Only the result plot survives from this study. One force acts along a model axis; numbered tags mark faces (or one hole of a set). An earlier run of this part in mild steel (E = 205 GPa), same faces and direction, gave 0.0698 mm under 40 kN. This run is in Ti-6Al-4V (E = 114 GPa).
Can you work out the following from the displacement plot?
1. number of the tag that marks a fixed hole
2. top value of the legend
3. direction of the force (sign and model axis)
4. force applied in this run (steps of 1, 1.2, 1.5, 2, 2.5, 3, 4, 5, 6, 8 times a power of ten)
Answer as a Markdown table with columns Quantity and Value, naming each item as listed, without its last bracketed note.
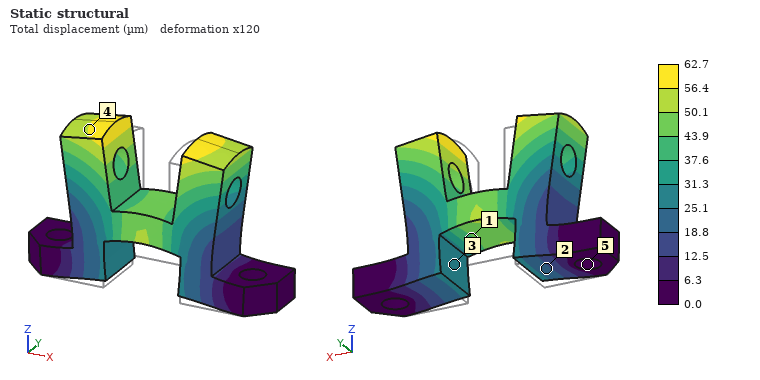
| Quantity | Value |
|---|---|
| number of the tag that marks a fixed hole | 5 |
| top value of the legend | 62.7 µm |
| direction of the force | +Z |
| force applied in this run | 20 kN |
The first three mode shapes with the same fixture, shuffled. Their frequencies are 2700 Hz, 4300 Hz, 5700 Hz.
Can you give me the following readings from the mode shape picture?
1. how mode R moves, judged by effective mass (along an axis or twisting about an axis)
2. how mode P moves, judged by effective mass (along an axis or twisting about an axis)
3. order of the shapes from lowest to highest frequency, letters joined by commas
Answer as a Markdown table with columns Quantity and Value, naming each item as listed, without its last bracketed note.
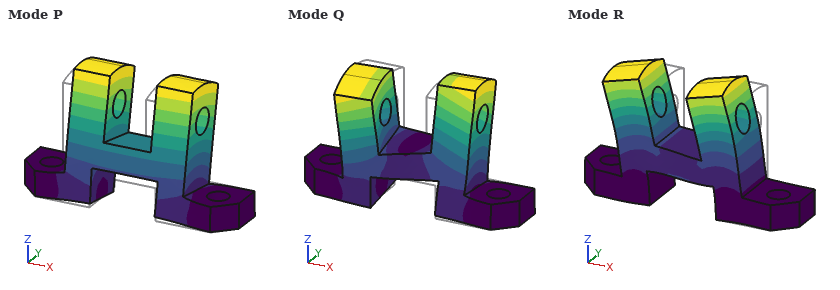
| Quantity | Value |
|---|---|
| how mode R moves, judged by effective mass | along X |
| how mode P moves, judged by effective mass | along Y |
| order of the shapes from lowest to highest frequency, letters joined by commas | P, Q, R |
